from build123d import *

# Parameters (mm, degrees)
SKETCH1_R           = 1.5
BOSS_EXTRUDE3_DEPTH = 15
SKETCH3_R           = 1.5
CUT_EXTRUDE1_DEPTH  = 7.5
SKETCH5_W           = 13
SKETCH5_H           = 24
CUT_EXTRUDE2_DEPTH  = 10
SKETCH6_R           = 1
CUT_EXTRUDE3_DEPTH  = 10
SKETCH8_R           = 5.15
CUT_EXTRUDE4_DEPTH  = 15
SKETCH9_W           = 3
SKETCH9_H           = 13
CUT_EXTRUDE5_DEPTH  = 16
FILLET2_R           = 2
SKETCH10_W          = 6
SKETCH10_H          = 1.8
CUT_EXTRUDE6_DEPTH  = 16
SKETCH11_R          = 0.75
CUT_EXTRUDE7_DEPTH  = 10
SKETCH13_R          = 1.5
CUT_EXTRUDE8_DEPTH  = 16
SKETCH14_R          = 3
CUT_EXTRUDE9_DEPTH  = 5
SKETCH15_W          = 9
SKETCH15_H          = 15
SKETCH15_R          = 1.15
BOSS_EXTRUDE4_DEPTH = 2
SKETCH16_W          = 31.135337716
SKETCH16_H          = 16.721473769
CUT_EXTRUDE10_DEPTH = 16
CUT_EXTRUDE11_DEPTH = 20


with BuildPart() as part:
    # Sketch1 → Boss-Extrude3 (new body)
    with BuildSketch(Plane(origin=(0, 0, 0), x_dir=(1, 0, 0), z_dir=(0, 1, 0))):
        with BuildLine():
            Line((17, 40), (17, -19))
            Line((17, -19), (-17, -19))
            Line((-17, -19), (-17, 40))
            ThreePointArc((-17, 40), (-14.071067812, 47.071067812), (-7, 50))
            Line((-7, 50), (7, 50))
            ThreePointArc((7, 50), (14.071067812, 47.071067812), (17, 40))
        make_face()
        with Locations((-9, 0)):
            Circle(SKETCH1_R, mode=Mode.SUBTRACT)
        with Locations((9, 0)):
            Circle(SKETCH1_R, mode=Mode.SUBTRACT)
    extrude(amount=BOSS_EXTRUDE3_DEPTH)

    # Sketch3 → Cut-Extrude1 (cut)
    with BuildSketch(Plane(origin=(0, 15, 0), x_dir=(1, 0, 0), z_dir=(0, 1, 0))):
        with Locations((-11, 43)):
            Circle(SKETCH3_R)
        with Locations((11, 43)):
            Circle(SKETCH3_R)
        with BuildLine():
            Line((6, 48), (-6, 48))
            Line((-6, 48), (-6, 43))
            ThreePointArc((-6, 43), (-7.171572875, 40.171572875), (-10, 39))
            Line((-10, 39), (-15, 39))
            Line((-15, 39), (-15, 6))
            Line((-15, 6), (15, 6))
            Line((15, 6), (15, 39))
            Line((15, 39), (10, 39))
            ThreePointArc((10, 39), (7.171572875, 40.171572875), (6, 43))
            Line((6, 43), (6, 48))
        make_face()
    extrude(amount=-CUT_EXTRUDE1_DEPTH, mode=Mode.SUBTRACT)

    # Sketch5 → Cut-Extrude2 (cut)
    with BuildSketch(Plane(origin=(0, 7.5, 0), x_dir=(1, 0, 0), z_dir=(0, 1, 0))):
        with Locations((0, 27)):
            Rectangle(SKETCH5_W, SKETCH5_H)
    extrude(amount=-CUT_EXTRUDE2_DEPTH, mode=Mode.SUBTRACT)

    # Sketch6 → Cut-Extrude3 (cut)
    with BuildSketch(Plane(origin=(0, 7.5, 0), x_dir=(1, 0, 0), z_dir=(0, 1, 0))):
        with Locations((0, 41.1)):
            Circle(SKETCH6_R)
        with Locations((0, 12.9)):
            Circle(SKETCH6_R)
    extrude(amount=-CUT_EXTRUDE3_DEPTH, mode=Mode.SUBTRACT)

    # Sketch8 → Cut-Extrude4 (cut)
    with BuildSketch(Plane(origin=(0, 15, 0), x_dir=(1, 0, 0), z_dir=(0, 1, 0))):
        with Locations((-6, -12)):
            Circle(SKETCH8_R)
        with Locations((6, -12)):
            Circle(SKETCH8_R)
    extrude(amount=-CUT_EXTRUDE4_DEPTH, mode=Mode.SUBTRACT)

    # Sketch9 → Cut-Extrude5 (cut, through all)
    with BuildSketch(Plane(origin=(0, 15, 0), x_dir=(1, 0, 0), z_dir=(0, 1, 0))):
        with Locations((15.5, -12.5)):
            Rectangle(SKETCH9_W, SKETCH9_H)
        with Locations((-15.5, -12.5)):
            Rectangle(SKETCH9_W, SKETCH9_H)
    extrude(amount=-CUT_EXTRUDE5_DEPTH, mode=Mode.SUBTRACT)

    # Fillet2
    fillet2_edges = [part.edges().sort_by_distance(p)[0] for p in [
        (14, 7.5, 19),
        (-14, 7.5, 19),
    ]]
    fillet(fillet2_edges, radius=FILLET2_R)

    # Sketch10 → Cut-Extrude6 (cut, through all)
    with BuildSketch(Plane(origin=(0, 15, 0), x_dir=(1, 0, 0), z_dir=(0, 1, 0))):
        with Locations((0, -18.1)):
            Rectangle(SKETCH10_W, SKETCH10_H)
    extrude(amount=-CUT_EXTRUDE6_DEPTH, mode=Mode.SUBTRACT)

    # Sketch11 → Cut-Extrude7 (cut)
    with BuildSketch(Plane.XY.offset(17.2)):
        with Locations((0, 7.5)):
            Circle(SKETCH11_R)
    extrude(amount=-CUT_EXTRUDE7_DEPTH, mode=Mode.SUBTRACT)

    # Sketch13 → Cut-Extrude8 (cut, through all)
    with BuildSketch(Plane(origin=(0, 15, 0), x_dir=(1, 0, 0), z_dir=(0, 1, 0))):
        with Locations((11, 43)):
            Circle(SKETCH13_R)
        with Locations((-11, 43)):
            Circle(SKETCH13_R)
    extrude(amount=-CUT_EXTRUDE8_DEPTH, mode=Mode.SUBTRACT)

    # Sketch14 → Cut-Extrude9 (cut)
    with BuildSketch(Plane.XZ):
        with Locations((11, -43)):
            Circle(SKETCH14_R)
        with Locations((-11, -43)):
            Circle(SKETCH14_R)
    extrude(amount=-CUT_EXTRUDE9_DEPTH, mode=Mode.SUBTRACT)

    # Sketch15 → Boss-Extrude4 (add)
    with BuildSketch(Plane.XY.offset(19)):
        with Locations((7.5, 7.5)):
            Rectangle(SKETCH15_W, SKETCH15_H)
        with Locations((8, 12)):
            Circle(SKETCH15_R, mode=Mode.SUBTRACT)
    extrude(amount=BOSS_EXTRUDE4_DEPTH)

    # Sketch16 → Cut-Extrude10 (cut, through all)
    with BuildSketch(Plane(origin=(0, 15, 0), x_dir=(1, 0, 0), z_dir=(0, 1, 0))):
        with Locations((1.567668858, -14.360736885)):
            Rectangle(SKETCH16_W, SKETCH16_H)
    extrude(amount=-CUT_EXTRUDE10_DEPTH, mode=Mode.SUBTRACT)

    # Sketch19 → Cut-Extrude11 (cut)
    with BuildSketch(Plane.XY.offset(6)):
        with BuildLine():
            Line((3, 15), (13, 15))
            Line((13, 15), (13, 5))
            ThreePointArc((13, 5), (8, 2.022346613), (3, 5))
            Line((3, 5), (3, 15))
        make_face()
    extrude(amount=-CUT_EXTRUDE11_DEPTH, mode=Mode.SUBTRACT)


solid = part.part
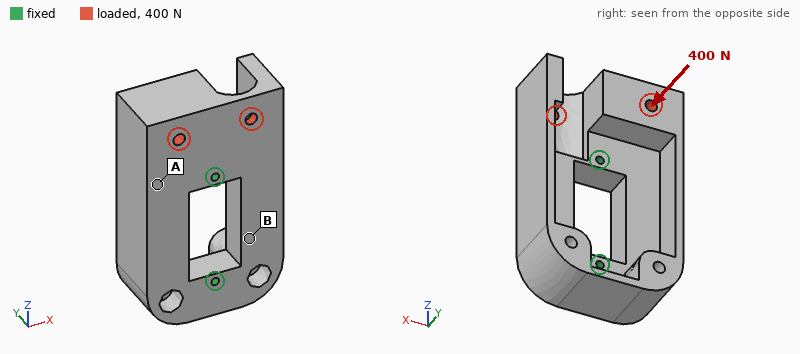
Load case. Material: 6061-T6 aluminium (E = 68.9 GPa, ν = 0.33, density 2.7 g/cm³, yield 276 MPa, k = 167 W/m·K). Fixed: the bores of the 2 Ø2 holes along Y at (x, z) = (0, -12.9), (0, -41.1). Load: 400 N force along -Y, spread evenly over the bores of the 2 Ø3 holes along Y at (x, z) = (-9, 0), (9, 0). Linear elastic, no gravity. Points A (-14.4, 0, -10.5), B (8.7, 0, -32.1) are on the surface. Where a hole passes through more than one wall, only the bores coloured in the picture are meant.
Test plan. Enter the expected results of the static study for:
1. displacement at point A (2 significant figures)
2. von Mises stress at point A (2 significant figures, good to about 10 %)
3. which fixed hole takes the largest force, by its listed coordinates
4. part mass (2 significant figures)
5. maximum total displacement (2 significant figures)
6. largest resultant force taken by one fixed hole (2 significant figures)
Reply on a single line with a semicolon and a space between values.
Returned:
12 µm; 8.4 MPa; (0, -12.9); 40 g; 28 µm; 470 N
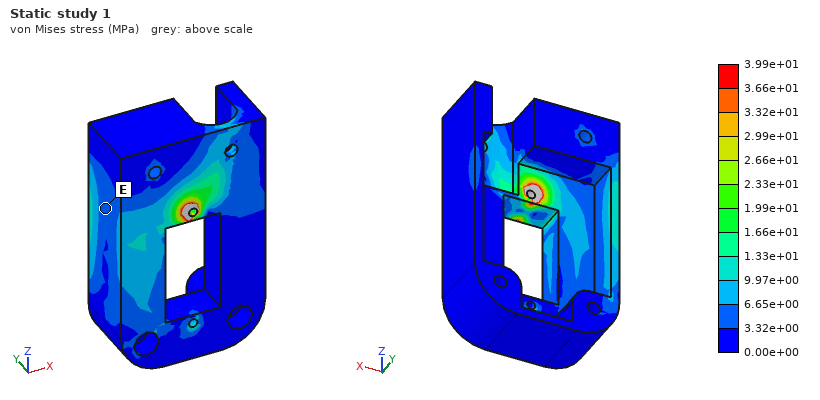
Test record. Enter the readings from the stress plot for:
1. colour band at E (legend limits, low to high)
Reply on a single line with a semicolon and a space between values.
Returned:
3.32e+00 to 6.65e+00 MPa
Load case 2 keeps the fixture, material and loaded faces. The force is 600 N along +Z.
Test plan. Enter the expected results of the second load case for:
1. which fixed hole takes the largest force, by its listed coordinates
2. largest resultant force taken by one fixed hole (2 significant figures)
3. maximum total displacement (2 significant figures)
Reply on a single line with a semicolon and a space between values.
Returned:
(0, -12.9); 470 N; 9.2 µm
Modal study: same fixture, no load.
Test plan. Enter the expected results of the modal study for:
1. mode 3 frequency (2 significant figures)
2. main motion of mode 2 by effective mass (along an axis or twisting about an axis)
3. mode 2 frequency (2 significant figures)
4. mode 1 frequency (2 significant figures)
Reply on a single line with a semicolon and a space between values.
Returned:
8700 Hz; along Y; 6800 Hz; 5700 Hz
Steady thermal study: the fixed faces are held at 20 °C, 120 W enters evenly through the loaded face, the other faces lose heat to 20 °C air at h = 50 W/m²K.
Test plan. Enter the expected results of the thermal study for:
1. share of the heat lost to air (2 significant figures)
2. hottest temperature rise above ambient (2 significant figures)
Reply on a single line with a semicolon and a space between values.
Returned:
9.0 %; 79 K
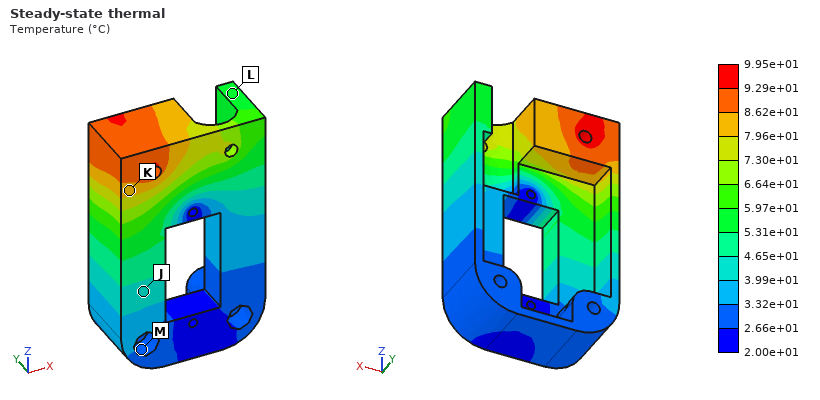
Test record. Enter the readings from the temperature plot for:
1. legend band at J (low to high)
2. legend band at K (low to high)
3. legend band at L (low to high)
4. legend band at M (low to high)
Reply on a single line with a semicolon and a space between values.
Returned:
3.99e+01 to 4.65e+01 °C; 7.96e+01 to 8.62e+01 °C; 5.31e+01 to 5.97e+01 °C; 2.66e+01 to 3.32e+01 °C
